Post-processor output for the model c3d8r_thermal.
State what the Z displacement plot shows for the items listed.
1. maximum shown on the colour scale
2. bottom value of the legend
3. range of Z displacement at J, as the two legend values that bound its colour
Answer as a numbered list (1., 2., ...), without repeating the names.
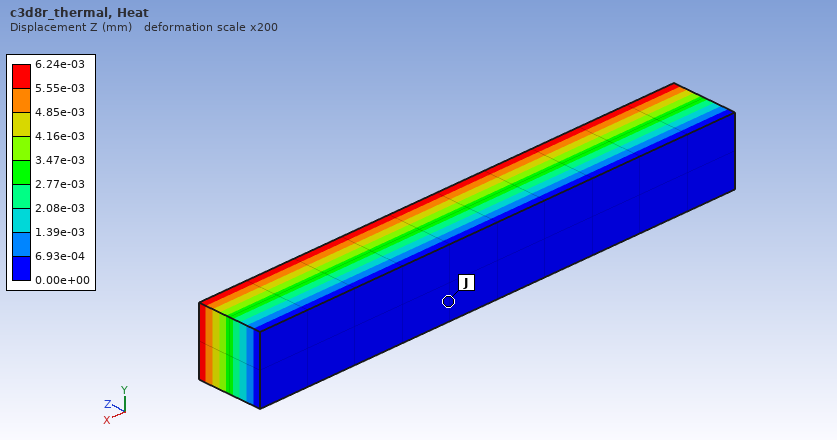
1. 6.24e-03 mm
2. 0.00e+00 mm
3. 0.00e+00 to 6.93e-04 mm
